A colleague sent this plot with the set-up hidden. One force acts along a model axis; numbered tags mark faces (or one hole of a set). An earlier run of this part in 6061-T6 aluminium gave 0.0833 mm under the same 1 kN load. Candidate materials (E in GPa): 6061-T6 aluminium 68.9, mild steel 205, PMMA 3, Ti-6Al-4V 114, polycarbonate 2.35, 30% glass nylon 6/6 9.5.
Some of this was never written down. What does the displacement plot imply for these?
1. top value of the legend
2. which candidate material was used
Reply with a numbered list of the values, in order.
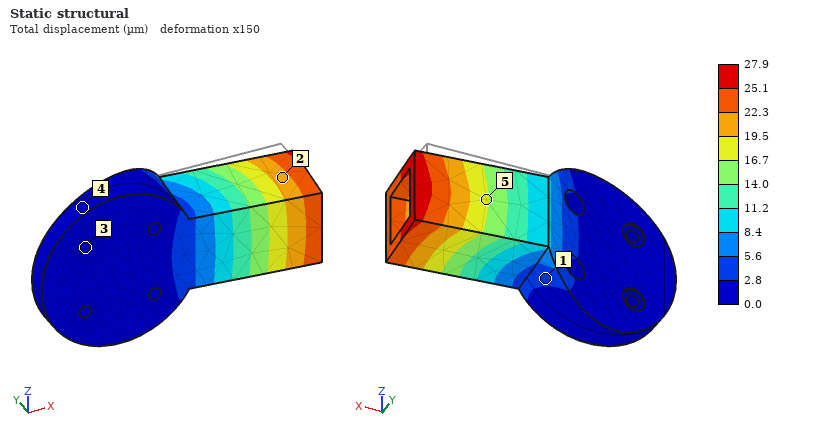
1. 27.9 µm
2. mild steel
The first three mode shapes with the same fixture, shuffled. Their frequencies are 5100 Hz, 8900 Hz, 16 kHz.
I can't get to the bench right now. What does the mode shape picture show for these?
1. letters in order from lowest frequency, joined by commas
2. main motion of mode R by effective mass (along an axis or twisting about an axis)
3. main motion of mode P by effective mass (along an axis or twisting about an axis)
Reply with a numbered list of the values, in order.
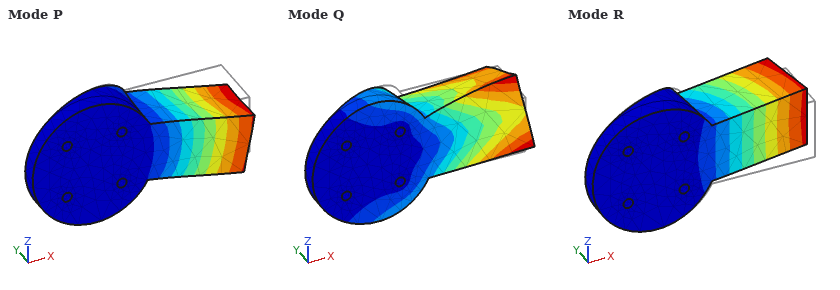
1. R, P, Q
2. along Y
3. along Z
